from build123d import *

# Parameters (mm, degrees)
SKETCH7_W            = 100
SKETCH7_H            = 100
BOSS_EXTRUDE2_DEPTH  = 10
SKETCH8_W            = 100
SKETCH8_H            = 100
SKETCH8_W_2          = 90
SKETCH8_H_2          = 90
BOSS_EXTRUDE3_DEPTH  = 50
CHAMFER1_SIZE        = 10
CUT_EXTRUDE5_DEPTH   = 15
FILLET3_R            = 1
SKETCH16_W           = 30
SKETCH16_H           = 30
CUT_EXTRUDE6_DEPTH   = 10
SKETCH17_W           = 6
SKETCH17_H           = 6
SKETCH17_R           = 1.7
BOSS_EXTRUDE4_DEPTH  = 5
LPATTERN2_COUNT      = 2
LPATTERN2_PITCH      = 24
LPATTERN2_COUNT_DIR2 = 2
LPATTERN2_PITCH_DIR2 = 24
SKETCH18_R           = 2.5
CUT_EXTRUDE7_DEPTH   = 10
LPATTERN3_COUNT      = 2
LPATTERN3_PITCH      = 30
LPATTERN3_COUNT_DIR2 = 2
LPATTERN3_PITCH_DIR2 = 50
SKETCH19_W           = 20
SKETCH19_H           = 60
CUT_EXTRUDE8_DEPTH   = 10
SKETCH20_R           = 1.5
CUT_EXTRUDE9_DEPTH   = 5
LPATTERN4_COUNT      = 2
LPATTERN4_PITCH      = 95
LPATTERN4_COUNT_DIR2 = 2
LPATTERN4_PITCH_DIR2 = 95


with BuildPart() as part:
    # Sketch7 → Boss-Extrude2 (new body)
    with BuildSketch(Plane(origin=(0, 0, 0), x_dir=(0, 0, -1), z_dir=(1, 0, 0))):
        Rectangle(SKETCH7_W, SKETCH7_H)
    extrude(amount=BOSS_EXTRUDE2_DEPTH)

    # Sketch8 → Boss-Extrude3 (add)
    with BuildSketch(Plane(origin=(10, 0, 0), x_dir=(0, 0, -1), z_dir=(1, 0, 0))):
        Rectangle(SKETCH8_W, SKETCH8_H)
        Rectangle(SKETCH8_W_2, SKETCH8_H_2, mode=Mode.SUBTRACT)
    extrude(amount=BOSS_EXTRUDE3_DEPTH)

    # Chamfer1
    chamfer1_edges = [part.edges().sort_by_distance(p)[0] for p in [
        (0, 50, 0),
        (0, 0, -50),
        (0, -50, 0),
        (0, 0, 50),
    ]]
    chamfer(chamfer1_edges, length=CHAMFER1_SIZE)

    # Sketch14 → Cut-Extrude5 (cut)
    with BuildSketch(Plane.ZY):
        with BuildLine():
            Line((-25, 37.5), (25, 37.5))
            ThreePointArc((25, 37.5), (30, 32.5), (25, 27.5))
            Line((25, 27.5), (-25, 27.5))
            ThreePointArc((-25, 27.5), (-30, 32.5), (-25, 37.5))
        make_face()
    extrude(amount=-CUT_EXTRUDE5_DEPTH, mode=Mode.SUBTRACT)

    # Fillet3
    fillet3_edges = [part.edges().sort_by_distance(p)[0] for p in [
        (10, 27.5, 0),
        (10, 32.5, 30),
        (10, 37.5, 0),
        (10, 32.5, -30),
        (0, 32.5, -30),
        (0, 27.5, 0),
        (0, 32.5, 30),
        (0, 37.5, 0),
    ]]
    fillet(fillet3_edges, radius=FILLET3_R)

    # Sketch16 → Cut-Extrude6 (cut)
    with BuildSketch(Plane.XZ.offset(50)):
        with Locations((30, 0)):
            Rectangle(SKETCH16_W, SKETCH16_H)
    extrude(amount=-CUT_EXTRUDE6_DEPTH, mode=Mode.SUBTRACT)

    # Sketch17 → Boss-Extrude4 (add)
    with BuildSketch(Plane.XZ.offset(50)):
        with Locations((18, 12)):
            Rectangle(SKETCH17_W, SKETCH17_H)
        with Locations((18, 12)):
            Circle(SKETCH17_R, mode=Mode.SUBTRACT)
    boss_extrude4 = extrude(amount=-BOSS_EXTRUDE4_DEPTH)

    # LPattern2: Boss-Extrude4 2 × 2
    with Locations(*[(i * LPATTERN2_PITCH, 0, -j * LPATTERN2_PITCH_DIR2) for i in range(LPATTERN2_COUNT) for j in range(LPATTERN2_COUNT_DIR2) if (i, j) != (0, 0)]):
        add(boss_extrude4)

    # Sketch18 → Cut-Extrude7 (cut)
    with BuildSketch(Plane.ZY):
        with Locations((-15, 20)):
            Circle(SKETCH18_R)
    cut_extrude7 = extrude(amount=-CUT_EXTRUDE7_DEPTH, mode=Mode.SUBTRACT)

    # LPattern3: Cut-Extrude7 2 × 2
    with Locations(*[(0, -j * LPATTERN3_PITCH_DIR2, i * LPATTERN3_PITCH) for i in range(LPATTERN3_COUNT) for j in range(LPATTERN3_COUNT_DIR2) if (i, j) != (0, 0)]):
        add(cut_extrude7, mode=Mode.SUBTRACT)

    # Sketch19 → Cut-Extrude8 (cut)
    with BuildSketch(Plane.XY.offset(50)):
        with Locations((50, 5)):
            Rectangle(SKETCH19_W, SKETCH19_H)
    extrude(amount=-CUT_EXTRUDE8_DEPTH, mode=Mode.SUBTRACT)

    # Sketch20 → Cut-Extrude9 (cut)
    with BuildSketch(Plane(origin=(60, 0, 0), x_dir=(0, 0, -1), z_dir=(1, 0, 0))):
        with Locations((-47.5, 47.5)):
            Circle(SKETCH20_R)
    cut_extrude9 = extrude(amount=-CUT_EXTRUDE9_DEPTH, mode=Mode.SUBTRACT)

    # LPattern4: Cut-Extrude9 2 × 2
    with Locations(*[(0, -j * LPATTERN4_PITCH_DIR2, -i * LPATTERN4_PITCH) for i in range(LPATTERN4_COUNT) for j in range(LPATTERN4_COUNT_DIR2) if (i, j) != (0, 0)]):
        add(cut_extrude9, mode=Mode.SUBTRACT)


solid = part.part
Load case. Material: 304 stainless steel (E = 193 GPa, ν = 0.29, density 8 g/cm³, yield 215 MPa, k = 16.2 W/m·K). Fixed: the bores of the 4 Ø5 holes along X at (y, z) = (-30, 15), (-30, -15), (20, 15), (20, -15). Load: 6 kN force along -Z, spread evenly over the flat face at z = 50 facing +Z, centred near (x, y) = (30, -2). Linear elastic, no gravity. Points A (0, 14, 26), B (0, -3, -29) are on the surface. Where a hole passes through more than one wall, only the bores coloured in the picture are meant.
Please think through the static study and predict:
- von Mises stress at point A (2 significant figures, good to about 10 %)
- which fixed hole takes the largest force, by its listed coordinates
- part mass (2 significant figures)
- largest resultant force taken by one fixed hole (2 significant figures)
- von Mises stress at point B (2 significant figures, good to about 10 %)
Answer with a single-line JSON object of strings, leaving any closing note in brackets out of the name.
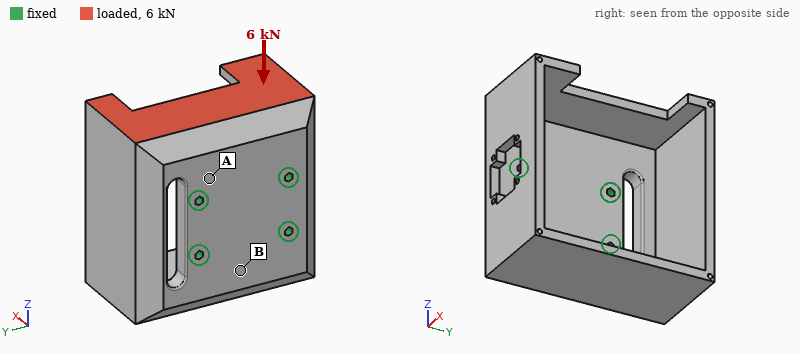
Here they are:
{"von Mises stress at point A": "34 MPa", "which fixed hole takes the largest force, by its listed coordinates": "(20, 15)", "part mass": "1.3 kg", "largest resultant force taken by one fixed hole": "2.7 kN", "von Mises stress at point B": "15 MPa"}
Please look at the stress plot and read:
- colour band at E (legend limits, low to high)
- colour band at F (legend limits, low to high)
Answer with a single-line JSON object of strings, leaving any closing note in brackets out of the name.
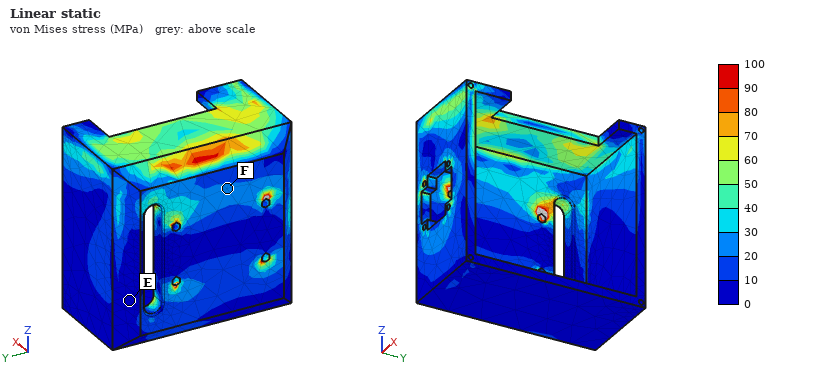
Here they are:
{"colour band at E": "0 to 10 MPa", "colour band at F": "20 to 30 MPa"}
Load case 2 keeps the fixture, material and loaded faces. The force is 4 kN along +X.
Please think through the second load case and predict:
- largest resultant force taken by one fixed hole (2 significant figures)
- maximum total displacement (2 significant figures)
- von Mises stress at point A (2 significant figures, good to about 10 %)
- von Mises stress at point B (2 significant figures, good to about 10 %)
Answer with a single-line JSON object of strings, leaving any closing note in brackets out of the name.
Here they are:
{"largest resultant force taken by one fixed hole": "3.2 kN", "maximum total displacement": "65 µm", "von Mises stress at point A": "55 MPa", "von Mises stress at point B": "8.7 MPa"}
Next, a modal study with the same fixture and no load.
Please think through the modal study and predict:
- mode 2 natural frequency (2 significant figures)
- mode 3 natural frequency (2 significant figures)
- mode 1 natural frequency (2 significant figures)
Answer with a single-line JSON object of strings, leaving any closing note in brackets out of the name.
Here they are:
{"mode 2 natural frequency": "1900 Hz", "mode 3 natural frequency": "2200 Hz", "mode 1 natural frequency": "1700 Hz"}
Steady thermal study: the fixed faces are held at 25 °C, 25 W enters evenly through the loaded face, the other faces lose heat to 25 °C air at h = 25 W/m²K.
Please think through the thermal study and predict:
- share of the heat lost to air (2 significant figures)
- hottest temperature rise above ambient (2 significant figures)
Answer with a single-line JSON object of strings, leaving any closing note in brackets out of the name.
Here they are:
{"share of the heat lost to air": "63 %", "hottest temperature rise above ambient": "58 K"}
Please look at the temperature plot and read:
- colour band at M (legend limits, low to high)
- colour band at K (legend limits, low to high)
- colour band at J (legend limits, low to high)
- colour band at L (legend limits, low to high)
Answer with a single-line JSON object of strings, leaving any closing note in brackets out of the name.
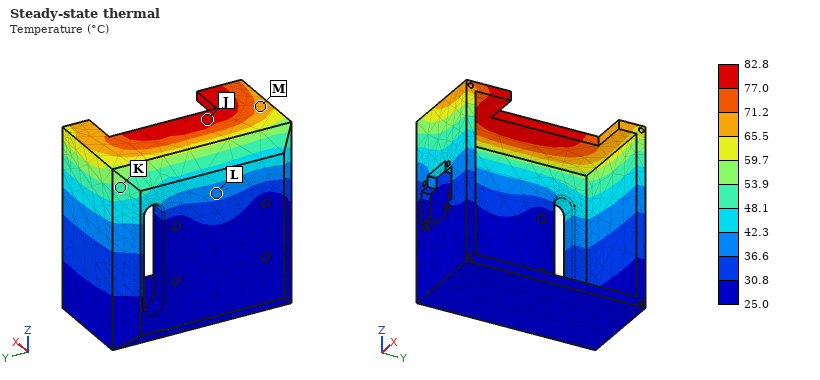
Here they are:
{"colour band at M": "65.5 to 71.2 °C", "colour band at K": "48.1 to 53.9 °C", "colour band at J": "77.0 to 82.8 °C", "colour band at L": "36.6 to 42.3 °C"}
